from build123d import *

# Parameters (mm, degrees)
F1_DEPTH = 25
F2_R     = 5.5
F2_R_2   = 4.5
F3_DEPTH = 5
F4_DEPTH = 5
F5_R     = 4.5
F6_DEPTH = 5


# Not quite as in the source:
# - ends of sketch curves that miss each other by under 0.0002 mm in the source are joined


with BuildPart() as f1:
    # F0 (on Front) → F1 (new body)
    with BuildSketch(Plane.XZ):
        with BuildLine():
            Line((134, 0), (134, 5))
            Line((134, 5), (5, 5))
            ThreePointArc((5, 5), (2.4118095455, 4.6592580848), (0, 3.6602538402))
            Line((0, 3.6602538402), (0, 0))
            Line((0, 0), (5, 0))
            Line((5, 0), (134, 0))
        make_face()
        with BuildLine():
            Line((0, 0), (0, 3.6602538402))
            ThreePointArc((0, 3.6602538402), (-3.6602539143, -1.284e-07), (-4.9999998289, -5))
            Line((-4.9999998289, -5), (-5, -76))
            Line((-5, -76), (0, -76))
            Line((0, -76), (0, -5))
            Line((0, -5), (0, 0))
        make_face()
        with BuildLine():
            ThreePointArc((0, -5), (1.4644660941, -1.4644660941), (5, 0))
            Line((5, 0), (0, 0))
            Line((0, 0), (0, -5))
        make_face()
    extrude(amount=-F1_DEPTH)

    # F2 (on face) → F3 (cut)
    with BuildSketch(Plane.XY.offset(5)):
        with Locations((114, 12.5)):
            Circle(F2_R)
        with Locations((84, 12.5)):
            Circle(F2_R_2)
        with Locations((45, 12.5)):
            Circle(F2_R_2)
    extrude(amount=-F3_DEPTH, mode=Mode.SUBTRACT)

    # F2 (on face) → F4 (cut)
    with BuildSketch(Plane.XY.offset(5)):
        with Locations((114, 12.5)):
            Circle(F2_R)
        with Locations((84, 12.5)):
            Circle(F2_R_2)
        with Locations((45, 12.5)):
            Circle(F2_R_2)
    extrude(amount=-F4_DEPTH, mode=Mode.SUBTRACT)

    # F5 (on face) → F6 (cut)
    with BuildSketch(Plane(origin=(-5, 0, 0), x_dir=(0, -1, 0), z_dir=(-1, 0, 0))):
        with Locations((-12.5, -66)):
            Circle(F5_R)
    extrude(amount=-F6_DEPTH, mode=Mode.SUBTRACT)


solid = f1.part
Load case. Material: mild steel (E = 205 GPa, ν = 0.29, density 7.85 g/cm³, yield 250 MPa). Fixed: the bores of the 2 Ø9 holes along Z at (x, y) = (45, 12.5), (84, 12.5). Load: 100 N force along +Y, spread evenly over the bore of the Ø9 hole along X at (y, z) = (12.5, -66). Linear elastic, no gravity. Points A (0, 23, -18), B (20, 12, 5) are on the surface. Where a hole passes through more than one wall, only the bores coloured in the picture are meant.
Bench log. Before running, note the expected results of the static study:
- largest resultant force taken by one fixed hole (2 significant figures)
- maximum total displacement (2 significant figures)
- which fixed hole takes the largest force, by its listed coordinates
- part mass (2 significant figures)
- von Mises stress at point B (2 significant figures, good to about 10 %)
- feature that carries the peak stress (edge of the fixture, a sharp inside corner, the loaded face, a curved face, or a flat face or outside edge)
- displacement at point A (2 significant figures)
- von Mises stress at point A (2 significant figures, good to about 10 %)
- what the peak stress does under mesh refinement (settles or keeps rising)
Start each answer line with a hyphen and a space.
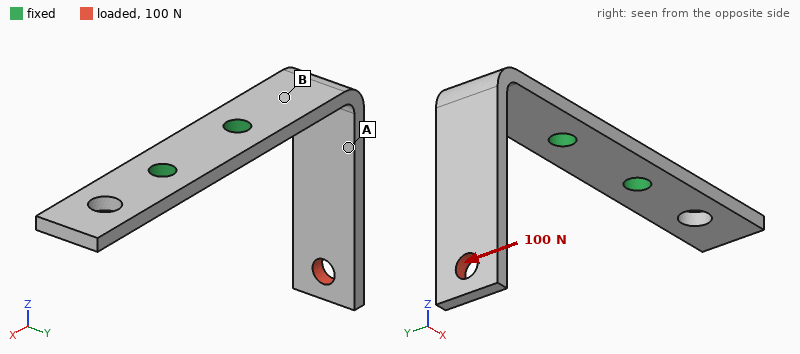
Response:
- 150 N
- 0.31 mm
- (45, 12.5)
- 200 g
- 61 MPa
- edge of the fixture
- 0.090 mm
- 10 MPa
- keeps rising
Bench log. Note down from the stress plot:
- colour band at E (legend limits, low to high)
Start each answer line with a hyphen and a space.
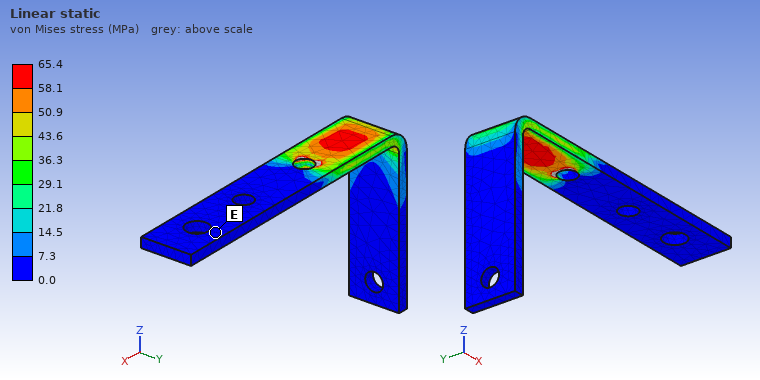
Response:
- 0.0 to 7.3 MPa
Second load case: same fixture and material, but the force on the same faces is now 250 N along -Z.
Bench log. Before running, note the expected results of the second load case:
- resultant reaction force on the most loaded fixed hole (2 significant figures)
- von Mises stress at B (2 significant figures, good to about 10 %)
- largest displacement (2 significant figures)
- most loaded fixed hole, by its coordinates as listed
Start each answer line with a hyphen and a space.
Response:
- 260 N
- 51 MPa
- 0.39 mm
- (45, 12.5)
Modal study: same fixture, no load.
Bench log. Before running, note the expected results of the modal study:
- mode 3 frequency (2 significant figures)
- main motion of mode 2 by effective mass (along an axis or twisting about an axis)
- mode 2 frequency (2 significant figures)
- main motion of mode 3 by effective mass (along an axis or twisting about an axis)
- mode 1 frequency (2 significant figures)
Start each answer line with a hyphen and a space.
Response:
- 1200 Hz
- along Y
- 540 Hz
- along Z
- 370 Hz
